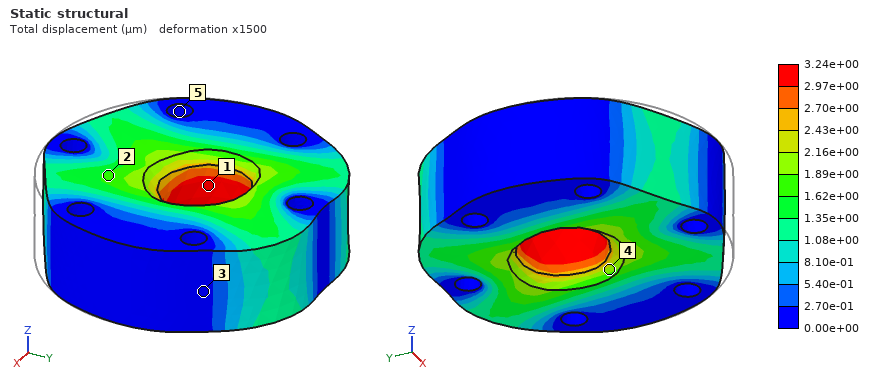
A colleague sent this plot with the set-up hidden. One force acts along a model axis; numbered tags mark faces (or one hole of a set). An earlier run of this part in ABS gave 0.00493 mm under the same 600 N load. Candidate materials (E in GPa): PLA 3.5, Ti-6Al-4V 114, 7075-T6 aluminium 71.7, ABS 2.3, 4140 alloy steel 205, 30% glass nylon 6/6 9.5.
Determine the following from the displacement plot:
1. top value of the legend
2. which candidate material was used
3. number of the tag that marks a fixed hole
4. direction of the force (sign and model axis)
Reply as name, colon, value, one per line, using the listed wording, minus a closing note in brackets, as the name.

top value of the legend: 3.24e+00 µm
which candidate material was used: PLA
number of the tag that marks a fixed hole: 5
direction of the force: +Y
